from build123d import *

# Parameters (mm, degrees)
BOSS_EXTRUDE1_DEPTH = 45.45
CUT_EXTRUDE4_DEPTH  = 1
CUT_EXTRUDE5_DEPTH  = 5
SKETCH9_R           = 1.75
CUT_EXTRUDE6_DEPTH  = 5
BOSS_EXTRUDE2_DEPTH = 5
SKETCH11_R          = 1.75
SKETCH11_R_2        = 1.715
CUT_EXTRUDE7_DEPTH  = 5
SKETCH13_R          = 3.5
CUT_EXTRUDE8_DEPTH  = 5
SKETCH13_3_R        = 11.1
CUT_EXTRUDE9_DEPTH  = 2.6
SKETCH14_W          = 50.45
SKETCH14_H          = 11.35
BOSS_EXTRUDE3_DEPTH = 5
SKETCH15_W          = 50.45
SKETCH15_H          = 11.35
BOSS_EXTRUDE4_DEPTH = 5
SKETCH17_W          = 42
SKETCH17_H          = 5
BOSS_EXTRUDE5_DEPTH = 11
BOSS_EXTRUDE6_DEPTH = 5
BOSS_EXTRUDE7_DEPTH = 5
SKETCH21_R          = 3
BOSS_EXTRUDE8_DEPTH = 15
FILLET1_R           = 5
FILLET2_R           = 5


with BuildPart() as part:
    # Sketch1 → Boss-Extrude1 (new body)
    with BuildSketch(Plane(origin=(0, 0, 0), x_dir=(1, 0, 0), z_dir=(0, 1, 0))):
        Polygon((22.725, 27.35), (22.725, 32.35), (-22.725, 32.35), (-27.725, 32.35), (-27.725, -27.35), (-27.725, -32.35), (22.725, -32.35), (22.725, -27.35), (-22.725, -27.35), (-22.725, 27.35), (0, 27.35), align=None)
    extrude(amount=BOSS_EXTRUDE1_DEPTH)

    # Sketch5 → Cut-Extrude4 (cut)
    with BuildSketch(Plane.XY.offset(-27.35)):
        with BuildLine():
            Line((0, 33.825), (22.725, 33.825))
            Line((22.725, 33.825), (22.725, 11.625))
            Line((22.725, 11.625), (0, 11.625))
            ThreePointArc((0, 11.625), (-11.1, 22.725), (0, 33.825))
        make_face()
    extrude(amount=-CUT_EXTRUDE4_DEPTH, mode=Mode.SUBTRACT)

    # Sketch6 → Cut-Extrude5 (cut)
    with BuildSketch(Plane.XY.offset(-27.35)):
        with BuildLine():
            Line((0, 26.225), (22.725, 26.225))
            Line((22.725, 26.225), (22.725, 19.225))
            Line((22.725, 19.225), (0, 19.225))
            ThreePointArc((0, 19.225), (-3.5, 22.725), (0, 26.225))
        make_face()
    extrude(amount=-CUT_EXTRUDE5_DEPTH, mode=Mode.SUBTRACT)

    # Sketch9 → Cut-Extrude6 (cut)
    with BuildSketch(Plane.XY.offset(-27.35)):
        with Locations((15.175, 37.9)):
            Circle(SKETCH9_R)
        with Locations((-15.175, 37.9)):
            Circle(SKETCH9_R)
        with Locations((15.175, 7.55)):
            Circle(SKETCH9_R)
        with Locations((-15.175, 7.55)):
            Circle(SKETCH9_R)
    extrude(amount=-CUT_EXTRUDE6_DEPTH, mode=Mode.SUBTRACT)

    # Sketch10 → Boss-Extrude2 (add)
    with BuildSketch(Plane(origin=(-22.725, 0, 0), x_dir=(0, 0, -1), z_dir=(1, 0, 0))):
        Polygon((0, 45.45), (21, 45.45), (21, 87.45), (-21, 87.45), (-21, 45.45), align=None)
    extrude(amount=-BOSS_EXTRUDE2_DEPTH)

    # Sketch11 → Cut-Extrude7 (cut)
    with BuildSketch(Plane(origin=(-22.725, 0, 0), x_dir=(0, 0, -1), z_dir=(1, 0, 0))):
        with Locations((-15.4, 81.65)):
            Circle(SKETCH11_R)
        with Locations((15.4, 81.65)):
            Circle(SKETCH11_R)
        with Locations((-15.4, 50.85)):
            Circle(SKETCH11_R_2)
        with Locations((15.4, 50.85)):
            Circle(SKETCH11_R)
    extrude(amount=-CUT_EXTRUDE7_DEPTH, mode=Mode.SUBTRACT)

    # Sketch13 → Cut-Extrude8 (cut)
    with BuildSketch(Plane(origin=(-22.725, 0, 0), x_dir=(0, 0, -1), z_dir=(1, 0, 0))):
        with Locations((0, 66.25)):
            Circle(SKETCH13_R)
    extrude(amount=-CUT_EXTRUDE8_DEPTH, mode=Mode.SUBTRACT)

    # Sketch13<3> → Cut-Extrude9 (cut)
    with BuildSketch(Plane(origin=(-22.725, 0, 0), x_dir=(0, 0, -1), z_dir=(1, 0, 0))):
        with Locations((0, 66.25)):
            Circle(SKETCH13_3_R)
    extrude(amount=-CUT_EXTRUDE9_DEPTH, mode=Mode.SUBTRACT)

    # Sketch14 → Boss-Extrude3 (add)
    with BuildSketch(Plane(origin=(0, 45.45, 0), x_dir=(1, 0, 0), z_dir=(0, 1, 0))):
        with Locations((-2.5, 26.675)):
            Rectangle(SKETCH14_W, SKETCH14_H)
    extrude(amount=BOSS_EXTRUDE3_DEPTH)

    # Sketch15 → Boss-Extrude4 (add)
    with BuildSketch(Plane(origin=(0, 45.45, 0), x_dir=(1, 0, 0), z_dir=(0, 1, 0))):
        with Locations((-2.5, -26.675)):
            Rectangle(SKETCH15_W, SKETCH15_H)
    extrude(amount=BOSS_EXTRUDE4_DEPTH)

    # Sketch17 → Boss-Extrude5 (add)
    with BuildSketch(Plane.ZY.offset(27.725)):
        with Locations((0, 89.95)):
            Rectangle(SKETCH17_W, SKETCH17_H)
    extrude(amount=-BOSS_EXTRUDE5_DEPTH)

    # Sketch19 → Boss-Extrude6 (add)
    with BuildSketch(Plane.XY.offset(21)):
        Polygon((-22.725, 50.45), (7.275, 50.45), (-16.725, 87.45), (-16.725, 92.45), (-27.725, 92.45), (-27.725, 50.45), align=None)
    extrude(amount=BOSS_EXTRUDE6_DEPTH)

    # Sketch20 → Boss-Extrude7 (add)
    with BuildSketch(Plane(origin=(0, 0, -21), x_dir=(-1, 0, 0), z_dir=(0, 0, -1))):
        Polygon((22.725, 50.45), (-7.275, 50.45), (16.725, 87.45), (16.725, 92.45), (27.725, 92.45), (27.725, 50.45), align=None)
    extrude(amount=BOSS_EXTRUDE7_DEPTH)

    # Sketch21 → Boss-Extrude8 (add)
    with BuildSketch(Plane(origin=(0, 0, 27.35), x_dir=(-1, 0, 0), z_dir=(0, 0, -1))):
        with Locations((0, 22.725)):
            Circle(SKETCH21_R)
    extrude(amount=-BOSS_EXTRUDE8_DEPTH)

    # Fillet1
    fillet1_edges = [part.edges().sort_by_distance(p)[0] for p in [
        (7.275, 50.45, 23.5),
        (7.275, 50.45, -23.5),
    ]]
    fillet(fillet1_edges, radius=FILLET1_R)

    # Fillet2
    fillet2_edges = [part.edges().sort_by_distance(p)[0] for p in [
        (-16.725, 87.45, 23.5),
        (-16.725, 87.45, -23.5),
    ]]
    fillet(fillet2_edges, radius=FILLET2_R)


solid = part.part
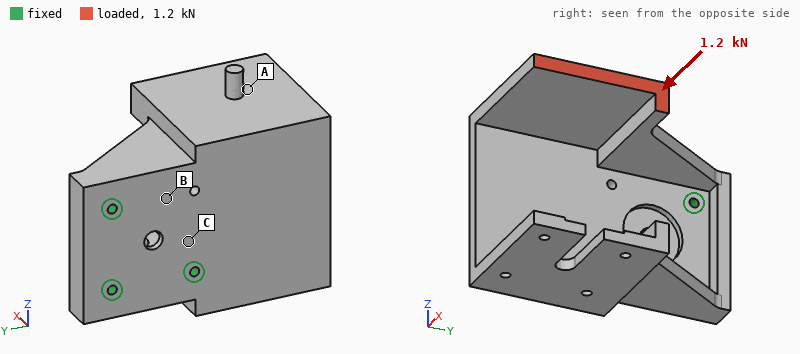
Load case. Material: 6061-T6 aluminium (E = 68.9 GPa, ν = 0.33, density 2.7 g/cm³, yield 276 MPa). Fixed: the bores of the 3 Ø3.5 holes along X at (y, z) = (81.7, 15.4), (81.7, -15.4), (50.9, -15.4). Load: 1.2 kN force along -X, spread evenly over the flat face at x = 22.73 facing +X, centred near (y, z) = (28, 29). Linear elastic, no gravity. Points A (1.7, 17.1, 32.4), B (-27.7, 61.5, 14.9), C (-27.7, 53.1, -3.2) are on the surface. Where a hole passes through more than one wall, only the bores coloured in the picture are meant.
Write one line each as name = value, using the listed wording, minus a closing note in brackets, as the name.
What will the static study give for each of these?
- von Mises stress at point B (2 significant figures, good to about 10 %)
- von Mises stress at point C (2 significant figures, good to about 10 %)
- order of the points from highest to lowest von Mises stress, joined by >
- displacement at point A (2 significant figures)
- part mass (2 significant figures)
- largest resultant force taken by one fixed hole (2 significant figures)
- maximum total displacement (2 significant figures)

von Mises stress at point B = 69 MPa
von Mises stress at point C = 100 MPa
order of the points from highest to lowest von Mises stress, joined by > = C > B > A
displacement at point A = 0.95 mm
part mass = 160 g
largest resultant force taken by one fixed hole = 1.2 kN
maximum total displacement = 1.3 mm
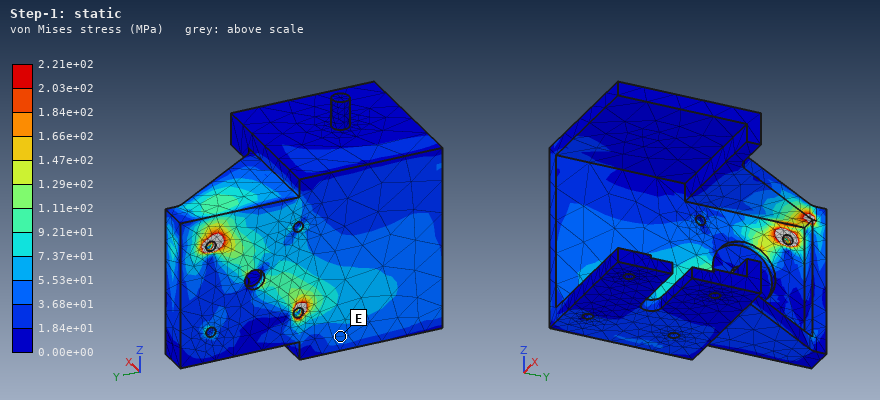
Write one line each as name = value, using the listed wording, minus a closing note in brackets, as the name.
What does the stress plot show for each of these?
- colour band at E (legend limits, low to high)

colour band at E = 3.68e+01 to 5.53e+01 MPa
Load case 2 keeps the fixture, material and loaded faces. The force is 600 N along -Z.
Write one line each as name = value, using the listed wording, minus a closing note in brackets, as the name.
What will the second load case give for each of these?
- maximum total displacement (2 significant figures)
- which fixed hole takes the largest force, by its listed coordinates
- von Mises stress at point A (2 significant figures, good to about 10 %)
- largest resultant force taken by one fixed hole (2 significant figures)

maximum total displacement = 1.2 mm
which fixed hole takes the largest force, by its listed coordinates = (50.9, -15.4)
von Mises stress at point A = 33 MPa
largest resultant force taken by one fixed hole = 1.0 kN
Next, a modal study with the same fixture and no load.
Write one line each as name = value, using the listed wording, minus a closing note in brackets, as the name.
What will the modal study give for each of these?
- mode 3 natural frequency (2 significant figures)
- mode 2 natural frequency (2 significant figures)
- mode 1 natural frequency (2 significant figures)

mode 3 natural frequency = 1600 Hz
mode 2 natural frequency = 1400 Hz
mode 1 natural frequency = 750 Hz
